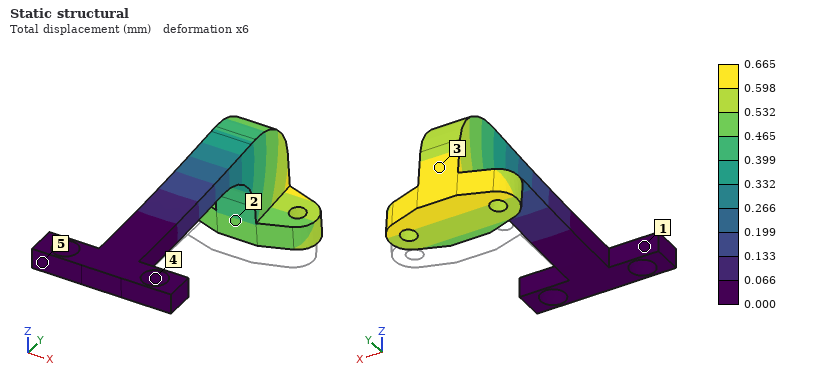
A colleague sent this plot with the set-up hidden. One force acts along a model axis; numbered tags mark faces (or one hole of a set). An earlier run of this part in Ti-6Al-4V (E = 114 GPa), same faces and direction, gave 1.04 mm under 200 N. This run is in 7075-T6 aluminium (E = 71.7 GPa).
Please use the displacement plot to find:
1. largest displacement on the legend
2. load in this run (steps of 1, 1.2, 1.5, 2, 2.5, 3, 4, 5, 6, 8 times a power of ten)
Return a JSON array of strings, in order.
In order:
["0.665 mm", "80 N"]
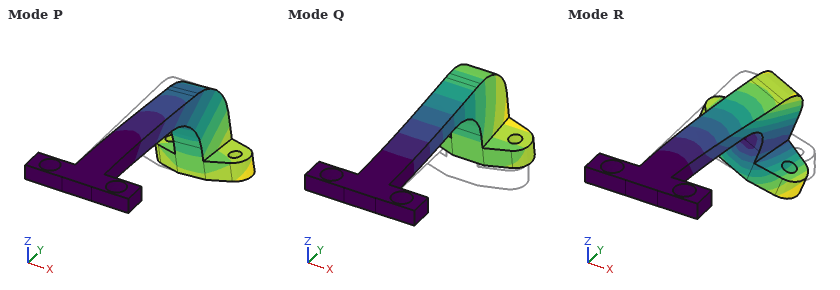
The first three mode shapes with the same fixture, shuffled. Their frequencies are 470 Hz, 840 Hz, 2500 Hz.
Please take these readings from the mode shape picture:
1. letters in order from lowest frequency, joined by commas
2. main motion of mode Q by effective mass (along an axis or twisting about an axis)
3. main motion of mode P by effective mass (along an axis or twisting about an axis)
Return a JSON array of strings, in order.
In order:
["Q, P, R", "along Z", "along X"]
